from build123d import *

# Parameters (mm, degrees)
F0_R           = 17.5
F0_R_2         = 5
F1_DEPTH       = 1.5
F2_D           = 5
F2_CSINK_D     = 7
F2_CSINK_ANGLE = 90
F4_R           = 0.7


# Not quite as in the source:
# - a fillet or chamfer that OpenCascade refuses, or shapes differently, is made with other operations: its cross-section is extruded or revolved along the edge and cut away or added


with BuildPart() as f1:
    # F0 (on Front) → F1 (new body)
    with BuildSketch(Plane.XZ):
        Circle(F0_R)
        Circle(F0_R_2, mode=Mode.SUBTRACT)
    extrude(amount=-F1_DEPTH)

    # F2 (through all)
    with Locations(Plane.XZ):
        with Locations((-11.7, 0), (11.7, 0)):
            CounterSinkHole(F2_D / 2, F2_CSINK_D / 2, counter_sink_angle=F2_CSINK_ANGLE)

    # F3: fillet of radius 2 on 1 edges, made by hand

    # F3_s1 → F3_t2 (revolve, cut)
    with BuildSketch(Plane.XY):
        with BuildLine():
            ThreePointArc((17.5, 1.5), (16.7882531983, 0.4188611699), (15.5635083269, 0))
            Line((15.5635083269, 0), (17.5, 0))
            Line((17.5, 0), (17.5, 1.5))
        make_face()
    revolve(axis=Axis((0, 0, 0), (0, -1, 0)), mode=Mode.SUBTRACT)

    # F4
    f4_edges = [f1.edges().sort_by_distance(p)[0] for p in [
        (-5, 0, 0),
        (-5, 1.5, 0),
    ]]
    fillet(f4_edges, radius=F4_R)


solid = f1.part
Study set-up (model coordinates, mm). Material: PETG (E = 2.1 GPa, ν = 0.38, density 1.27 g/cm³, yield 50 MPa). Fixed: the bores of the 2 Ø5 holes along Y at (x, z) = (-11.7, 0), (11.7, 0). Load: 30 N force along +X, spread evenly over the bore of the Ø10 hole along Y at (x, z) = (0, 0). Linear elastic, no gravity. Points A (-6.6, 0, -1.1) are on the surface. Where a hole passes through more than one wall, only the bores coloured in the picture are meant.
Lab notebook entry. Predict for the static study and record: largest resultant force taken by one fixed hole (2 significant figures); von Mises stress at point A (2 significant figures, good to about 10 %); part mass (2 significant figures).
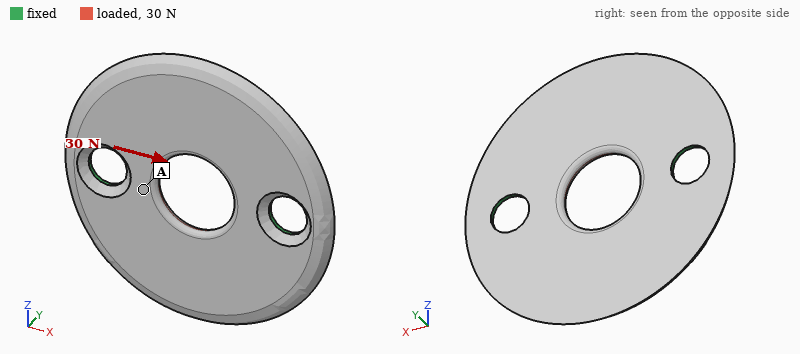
15 N
0.77 MPa
1.5 g
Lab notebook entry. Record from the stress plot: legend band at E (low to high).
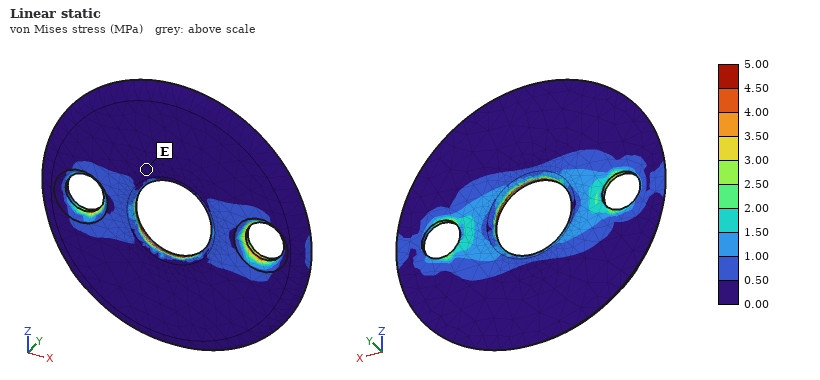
0.00 to 0.50 MPa
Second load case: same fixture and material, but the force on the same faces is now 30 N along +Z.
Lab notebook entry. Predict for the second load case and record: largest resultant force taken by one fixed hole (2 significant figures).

15 N
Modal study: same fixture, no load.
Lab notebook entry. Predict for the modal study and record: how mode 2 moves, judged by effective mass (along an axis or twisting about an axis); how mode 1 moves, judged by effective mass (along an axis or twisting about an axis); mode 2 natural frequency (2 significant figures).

along Y
twisting about X
1200 Hz
